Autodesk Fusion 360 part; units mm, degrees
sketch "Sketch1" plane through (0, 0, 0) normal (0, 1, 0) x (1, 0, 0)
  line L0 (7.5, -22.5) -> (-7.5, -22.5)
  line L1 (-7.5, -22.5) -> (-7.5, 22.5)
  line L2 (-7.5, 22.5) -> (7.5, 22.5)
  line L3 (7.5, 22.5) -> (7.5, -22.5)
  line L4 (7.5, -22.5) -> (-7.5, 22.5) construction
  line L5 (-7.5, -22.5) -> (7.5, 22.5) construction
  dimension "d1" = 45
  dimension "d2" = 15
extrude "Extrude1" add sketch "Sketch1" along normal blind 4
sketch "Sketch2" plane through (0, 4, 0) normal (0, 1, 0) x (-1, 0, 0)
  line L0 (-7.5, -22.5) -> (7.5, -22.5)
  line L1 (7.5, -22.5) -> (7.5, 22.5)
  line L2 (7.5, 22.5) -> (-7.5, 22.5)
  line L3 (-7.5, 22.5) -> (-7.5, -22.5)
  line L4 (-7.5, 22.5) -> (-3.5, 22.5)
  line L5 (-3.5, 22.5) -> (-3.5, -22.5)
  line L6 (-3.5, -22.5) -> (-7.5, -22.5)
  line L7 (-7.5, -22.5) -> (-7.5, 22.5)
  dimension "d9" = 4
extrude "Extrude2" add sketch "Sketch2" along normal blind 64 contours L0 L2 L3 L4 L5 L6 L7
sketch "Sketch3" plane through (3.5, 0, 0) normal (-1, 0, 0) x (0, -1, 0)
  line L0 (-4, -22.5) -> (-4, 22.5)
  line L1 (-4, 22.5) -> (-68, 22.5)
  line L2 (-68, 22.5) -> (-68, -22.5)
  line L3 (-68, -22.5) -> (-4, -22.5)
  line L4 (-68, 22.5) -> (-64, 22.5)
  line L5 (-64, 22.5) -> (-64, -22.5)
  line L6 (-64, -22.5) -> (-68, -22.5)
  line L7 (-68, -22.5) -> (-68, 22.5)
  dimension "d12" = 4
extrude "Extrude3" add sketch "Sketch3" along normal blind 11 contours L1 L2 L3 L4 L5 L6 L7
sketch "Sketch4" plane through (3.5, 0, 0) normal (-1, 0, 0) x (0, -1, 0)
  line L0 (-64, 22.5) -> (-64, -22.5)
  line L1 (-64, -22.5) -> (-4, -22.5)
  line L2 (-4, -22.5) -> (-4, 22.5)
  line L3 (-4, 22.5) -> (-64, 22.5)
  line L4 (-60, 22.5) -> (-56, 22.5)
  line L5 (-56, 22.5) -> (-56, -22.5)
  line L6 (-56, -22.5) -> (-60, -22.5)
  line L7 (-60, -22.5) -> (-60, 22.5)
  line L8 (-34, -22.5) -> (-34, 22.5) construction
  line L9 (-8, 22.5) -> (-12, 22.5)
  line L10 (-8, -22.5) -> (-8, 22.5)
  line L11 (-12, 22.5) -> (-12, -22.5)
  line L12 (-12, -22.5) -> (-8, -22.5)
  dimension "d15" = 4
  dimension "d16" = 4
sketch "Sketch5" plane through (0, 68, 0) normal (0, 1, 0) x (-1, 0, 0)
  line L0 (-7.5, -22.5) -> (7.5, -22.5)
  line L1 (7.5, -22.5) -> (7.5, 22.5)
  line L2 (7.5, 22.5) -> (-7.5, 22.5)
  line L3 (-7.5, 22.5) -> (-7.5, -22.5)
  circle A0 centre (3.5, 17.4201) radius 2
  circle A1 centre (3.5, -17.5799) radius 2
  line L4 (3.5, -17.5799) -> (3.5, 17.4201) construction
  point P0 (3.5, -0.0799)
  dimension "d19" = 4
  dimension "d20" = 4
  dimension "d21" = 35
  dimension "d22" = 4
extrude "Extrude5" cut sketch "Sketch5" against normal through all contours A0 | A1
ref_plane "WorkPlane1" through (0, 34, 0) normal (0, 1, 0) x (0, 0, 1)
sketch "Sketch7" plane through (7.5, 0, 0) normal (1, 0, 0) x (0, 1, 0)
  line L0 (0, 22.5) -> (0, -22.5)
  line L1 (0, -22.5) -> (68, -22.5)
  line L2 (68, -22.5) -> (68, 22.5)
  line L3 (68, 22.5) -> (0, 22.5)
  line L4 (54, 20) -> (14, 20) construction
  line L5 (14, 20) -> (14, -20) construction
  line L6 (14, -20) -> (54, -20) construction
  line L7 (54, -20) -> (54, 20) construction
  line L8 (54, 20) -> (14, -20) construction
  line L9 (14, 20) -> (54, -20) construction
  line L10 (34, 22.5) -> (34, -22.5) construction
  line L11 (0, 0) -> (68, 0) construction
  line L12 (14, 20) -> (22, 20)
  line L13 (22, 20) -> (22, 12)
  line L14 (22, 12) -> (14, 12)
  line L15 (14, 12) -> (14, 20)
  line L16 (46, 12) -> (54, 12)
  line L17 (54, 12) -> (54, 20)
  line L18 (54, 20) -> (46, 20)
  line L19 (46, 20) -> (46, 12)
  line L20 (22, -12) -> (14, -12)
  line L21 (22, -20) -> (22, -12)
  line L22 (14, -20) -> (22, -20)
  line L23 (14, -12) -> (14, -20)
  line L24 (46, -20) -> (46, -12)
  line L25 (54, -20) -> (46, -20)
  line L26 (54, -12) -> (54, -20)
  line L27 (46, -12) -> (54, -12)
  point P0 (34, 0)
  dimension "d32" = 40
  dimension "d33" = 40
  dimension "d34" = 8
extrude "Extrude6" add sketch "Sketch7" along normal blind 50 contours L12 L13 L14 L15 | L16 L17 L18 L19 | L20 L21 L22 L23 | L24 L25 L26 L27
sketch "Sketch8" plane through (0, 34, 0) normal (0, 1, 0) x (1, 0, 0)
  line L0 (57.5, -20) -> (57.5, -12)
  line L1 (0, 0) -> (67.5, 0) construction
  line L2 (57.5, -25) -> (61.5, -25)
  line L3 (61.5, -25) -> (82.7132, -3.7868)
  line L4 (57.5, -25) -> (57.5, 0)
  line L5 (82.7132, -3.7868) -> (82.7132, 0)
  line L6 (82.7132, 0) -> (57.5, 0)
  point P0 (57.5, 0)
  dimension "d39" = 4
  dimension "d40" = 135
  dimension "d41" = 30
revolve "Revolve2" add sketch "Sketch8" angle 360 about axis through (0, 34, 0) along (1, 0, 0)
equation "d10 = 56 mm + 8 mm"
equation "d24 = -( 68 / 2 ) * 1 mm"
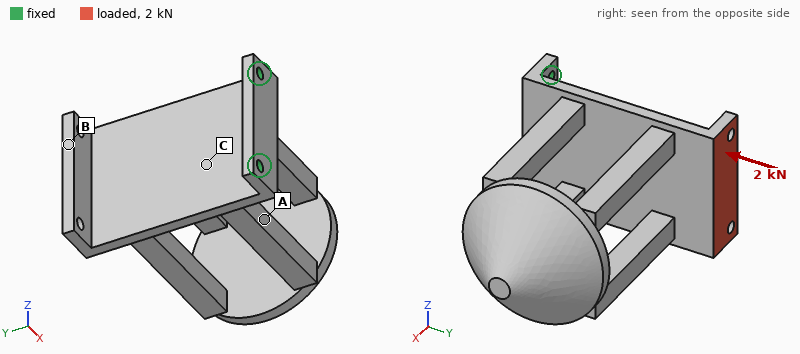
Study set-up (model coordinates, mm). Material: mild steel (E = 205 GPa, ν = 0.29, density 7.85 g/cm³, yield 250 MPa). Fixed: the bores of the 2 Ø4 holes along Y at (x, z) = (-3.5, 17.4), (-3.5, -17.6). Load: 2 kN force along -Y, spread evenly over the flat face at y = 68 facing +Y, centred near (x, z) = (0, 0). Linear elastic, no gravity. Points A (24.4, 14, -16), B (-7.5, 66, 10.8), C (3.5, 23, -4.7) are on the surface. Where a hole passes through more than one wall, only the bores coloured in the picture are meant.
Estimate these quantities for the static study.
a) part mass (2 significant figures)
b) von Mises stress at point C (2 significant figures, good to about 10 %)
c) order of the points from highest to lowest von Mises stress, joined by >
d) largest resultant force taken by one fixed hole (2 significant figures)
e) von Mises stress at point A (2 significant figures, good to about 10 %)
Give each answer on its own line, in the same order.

420 g
38 MPa
C > A > B
1.0 kN
24 MPa
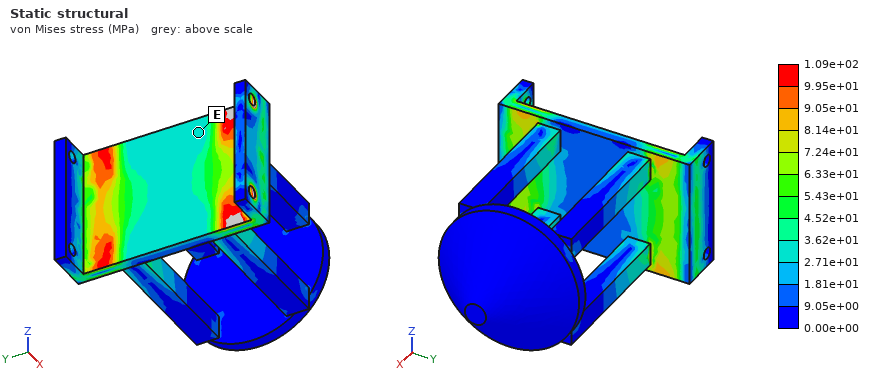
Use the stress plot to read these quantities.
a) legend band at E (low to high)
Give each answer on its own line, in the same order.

2.71e+01 to 3.62e+01 MPa
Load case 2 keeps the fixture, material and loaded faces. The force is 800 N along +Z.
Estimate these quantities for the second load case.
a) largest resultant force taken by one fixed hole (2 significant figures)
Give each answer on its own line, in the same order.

1.5 kN
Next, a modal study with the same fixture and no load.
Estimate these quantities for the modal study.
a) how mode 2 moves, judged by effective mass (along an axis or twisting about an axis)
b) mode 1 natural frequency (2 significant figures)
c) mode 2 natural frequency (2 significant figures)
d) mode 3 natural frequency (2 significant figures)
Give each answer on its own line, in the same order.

along Z
190 Hz
630 Hz
1600 Hz
